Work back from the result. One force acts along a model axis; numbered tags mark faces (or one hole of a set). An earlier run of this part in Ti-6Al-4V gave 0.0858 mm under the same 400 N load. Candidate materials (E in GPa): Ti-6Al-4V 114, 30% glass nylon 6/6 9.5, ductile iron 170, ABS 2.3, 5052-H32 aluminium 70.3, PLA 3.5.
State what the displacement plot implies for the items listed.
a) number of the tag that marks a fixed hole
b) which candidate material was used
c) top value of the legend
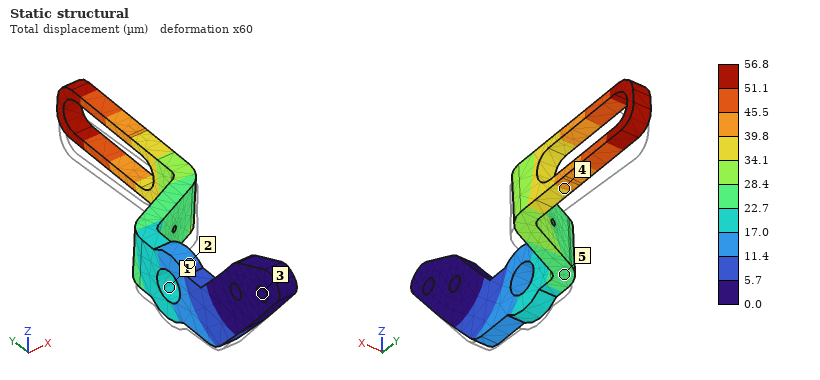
3
ductile iron
56.8 µm
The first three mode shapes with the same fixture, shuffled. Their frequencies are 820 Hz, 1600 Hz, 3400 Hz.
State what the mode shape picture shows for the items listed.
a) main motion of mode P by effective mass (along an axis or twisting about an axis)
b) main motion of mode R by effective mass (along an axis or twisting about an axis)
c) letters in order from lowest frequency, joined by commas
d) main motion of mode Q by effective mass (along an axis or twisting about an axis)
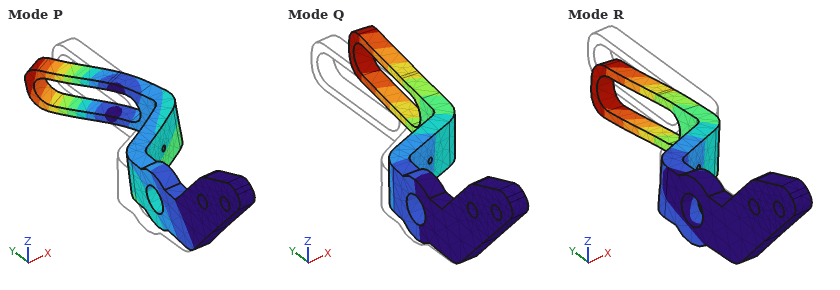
along X
along Z
Q, R, P
along X
